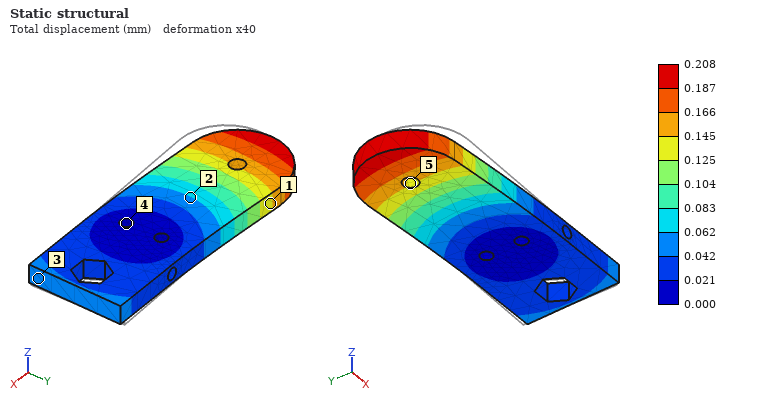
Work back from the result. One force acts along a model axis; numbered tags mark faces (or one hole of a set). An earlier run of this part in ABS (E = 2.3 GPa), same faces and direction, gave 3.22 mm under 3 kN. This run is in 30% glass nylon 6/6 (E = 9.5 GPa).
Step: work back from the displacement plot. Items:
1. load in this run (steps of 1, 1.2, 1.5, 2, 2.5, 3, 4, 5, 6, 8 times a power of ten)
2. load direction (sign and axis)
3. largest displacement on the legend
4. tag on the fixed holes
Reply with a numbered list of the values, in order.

1. 800 N
2. +Y
3. 0.208 mm
4. 4
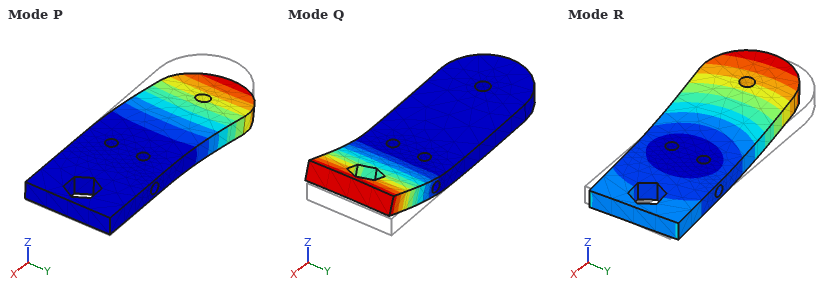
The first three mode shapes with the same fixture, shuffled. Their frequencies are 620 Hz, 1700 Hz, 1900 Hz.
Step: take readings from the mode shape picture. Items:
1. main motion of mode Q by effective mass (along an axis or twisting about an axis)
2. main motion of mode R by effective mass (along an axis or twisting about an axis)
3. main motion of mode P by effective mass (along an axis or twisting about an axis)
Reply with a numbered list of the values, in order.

1. along Z
2. along Y
3. along Z
